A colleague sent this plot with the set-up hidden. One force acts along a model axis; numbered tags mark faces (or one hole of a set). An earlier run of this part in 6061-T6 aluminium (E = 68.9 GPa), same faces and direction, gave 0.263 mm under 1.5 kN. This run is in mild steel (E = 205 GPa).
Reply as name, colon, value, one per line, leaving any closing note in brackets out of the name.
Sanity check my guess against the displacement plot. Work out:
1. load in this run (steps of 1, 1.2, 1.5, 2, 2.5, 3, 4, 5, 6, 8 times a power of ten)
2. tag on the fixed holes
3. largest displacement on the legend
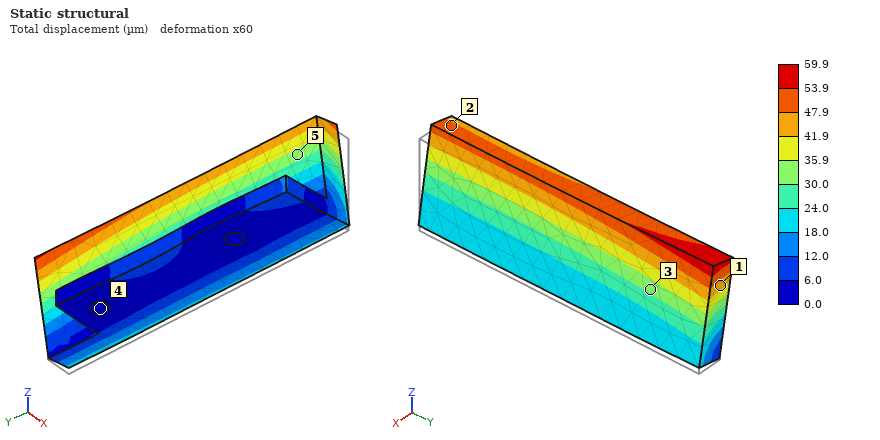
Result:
load in this run: 1 kN
tag on the fixed holes: 4
largest displacement on the legend: 59.9 µm
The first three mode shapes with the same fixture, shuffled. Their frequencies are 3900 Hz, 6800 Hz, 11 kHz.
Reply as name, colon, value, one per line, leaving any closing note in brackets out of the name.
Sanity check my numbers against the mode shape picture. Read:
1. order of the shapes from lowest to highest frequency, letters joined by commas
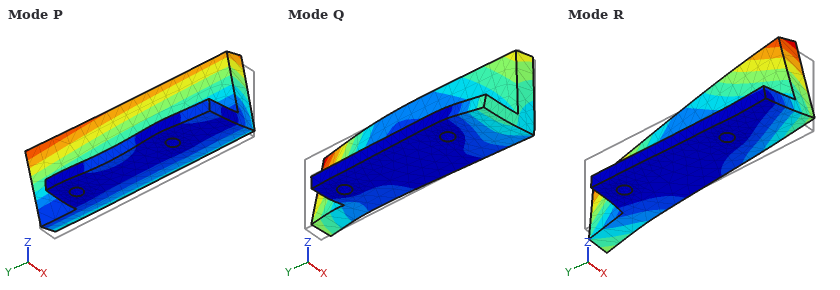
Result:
order of the shapes from lowest to highest frequency, letters joined by commas: P, R, Q
